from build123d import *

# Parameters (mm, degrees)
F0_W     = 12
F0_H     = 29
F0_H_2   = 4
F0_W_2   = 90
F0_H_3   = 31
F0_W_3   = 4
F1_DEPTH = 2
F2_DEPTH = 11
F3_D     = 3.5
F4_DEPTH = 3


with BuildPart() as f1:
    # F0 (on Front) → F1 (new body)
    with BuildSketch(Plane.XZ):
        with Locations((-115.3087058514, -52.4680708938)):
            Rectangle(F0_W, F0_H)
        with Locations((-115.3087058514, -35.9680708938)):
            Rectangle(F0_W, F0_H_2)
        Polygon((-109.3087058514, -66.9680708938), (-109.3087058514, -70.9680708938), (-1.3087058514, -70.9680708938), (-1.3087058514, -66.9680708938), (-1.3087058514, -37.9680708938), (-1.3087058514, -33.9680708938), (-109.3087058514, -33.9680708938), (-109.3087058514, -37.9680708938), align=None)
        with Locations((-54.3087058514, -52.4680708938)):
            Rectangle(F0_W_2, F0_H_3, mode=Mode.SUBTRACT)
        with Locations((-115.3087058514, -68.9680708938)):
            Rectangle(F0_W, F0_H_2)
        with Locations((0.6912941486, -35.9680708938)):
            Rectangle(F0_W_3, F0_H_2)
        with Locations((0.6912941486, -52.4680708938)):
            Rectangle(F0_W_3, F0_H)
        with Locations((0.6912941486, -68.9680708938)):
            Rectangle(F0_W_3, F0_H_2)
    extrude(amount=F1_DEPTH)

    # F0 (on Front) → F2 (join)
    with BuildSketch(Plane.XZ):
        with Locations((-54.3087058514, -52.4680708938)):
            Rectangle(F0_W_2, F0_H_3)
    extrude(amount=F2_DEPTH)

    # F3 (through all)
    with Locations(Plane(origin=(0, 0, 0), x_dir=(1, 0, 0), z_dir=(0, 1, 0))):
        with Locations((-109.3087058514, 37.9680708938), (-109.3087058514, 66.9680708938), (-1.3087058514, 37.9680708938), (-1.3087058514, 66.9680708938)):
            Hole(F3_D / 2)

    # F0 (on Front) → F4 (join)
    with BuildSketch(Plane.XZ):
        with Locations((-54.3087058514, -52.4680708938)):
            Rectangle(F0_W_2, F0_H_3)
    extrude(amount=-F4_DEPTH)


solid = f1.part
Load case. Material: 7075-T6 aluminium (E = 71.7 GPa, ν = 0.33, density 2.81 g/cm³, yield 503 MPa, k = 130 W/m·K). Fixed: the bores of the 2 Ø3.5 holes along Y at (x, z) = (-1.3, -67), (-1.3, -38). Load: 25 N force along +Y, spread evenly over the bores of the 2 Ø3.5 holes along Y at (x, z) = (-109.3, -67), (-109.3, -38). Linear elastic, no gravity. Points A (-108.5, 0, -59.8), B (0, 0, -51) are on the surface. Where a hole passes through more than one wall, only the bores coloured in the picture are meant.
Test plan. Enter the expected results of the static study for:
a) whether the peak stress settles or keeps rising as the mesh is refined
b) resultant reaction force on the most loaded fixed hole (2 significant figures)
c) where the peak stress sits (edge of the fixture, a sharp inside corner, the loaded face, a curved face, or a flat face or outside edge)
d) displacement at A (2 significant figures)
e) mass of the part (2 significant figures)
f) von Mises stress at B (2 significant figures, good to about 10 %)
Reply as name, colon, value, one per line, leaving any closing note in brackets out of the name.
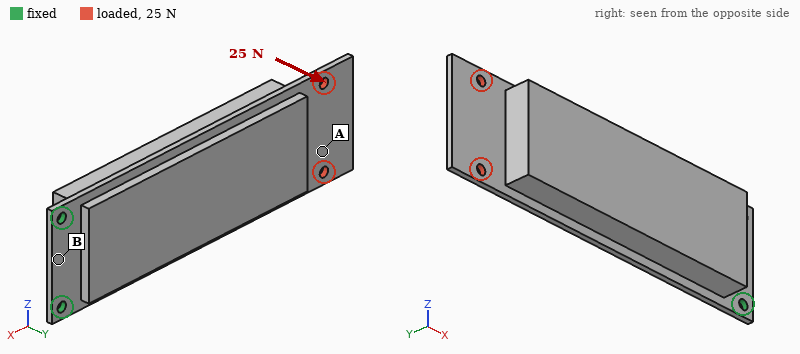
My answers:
whether the peak stress settles or keeps rising as the mesh is refined: keeps rising
resultant reaction force on the most loaded fixed hole: 13 N
where the peak stress sits: edge of the fixture
displacement at A: 1.3 mm
mass of the part: 120 g
von Mises stress at B: 34 MPa
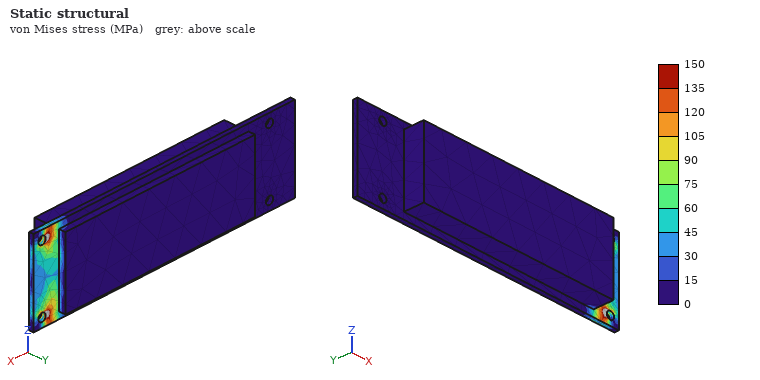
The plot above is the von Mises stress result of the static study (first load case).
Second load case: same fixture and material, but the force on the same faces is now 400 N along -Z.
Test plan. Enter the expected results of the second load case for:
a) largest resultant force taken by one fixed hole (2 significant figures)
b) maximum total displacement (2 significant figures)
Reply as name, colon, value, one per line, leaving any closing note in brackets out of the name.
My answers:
largest resultant force taken by one fixed hole: 1.5 kN
maximum total displacement: 0.16 mm
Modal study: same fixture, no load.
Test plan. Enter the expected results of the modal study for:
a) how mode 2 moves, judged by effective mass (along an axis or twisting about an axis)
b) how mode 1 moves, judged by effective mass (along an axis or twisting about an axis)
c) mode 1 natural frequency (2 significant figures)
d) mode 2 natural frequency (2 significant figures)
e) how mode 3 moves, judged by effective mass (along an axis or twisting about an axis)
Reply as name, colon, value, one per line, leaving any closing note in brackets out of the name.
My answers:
how mode 2 moves, judged by effective mass: along Z
how mode 1 moves, judged by effective mass: along Y
mode 1 natural frequency: 110 Hz
mode 2 natural frequency: 1500 Hz
how mode 3 moves, judged by effective mass: twisting about X
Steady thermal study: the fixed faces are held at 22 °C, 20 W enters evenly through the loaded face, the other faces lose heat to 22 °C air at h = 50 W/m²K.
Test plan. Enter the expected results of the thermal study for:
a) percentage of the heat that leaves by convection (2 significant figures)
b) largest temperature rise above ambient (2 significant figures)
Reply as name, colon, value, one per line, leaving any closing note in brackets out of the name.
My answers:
percentage of the heat that leaves by convection: 63 %
largest temperature rise above ambient: 57 K
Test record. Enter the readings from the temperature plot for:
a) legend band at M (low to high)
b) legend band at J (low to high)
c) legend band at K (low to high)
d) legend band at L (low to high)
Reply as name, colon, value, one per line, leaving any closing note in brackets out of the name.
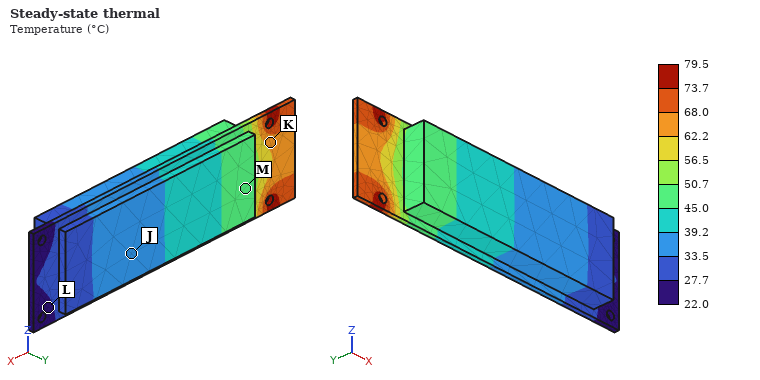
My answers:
legend band at M: 45.0 to 50.7 °C
legend band at J: 33.5 to 39.2 °C
legend band at K: 62.2 to 68.0 °C
legend band at L: 22.0 to 27.7 °C
